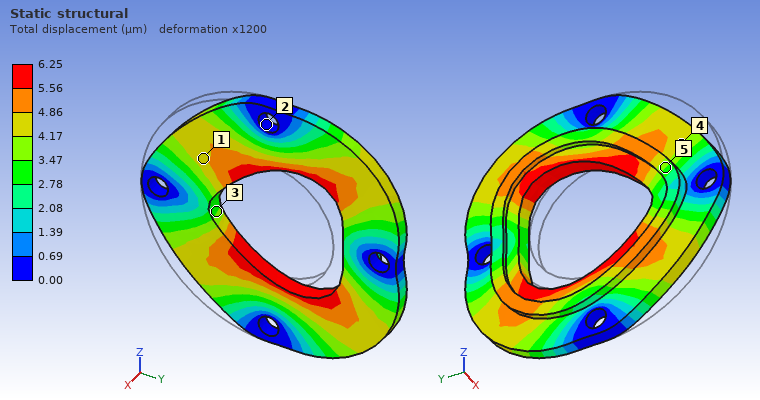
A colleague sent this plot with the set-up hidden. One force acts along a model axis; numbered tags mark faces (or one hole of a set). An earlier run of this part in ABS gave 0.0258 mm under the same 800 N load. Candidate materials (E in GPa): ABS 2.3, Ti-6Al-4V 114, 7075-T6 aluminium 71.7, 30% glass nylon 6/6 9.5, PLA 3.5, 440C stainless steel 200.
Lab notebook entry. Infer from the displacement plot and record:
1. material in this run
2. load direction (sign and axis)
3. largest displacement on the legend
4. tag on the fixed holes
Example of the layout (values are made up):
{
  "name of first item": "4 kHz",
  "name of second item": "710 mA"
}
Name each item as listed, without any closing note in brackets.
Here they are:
{
  "material in this run": "30% glass nylon 6/6",
  "load direction": "+Y",
  "largest displacement on the legend": "6.25 µm",
  "tag on the fixed holes": "2"
}
